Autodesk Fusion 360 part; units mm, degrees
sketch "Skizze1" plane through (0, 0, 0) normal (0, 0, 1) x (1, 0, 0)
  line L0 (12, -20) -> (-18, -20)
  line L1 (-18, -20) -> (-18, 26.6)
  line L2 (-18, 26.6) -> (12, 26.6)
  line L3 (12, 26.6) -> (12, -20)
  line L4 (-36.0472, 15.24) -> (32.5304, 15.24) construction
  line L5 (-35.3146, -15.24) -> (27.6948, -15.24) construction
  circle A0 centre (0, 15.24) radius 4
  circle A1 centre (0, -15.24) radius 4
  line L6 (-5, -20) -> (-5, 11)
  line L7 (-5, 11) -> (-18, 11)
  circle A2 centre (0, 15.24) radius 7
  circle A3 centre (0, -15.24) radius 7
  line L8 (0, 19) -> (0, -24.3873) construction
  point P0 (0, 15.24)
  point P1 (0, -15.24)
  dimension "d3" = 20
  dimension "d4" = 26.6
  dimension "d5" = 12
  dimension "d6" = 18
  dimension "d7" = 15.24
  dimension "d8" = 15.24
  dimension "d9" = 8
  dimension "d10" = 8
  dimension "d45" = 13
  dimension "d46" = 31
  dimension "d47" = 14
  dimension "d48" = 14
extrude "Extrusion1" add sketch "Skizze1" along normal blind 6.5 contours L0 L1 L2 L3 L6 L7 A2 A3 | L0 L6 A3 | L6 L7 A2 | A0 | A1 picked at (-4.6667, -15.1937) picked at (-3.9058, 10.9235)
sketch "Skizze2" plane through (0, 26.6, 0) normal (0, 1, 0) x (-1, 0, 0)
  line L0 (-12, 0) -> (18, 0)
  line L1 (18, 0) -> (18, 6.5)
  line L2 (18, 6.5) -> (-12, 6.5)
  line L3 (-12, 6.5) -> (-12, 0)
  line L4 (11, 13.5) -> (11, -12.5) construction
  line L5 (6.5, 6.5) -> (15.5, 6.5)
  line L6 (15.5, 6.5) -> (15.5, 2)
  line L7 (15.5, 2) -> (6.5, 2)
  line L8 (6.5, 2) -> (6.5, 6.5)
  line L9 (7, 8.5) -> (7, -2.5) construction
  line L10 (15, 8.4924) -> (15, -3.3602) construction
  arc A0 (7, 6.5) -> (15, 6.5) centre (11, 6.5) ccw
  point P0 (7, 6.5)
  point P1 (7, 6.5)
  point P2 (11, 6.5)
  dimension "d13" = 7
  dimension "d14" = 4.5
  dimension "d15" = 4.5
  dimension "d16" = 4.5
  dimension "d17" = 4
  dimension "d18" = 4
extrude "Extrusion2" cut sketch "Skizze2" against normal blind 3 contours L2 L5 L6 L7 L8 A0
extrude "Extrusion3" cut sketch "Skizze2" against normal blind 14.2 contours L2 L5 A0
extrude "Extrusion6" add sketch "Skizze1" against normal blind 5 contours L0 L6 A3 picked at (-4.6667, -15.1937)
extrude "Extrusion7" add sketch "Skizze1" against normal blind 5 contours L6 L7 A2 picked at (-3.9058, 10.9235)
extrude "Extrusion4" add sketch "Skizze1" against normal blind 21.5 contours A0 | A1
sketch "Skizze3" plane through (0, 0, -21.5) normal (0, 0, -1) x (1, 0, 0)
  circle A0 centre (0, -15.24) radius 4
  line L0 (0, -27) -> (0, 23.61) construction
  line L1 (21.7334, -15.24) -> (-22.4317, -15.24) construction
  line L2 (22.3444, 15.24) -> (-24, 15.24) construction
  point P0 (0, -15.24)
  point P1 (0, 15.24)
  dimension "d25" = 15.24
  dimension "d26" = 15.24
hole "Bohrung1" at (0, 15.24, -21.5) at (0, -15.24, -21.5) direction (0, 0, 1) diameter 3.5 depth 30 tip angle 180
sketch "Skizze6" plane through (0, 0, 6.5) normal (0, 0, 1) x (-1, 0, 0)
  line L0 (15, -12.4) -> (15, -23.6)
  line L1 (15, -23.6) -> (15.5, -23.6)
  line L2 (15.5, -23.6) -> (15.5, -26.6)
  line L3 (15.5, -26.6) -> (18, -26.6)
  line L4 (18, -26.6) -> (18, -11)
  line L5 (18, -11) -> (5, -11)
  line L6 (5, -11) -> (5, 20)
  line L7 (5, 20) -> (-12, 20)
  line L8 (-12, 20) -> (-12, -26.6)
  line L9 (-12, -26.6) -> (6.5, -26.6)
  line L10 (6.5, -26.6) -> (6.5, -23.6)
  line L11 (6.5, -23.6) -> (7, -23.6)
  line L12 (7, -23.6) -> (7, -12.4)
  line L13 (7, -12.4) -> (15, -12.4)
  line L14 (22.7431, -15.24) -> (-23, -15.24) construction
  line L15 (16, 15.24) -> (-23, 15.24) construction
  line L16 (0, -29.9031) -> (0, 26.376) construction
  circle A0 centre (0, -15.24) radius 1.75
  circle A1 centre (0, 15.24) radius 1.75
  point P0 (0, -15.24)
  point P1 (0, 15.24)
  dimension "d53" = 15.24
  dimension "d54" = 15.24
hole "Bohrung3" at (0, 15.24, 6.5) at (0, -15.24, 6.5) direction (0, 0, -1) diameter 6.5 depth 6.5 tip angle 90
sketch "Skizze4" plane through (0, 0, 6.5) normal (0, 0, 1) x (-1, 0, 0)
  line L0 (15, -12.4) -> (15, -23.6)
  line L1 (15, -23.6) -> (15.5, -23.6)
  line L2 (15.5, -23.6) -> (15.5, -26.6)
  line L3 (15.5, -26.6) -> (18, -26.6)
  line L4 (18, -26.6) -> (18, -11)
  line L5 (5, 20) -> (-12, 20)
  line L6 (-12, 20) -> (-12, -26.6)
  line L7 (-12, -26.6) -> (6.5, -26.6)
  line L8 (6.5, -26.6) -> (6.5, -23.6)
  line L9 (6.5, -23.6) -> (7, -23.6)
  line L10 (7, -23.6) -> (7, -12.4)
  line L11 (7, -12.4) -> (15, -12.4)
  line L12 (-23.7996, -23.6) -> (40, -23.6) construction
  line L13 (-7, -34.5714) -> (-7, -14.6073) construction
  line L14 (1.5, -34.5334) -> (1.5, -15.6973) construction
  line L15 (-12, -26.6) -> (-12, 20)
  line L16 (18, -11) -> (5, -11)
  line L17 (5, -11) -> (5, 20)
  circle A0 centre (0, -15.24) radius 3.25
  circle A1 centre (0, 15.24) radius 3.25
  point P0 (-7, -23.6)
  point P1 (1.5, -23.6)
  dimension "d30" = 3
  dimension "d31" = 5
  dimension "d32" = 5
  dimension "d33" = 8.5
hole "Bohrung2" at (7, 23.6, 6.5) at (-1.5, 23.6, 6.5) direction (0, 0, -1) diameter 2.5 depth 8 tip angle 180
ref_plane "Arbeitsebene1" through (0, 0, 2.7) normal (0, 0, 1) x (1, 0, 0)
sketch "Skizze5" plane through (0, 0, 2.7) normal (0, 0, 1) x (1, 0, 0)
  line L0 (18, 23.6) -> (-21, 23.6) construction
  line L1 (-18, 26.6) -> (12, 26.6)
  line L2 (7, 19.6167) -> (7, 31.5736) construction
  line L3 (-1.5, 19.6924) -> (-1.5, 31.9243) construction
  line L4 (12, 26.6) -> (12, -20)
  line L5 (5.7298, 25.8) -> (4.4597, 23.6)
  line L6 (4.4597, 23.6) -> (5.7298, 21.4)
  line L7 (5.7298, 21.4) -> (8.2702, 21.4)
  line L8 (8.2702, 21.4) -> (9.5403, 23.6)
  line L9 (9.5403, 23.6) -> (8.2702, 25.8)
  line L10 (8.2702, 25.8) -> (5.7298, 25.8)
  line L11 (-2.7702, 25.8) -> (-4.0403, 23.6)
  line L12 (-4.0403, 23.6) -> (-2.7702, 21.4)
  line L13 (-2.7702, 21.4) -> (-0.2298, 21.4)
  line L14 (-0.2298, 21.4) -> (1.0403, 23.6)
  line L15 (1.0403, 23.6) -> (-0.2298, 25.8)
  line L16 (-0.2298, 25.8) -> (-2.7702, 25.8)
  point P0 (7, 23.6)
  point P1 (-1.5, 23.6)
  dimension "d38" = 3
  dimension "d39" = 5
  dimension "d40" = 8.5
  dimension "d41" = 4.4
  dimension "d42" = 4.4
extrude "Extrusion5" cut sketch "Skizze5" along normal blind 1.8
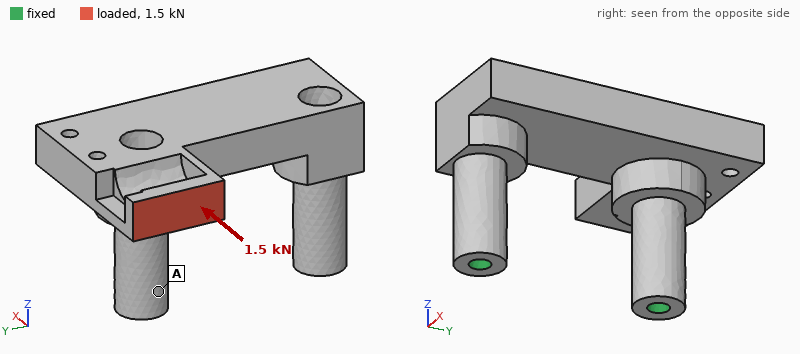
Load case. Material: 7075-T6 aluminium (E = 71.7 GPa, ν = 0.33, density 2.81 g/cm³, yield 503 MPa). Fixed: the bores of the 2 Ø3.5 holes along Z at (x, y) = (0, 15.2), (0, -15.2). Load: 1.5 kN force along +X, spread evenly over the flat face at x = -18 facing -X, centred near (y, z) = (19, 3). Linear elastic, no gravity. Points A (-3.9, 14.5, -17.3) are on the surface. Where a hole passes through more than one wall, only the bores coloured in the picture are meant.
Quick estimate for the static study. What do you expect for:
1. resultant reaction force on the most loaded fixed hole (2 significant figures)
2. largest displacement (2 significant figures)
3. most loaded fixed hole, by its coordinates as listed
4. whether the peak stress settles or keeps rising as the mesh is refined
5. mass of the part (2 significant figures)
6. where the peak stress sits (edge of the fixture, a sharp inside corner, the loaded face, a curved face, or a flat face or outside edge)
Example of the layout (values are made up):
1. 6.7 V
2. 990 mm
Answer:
1. 1.5 kN
2. 0.11 mm
3. (0, 15.2)
4. keeps rising
5. 23 g
6. edge of the fixture
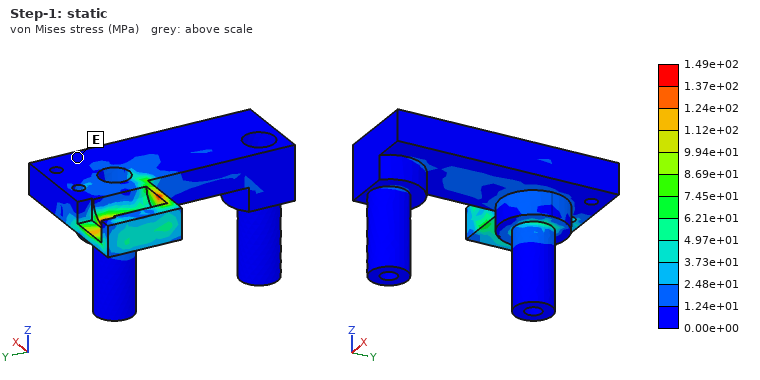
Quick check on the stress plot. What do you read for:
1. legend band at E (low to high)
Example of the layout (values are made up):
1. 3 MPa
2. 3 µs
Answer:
1. 0.00e+00 to 1.24e+01 MPa
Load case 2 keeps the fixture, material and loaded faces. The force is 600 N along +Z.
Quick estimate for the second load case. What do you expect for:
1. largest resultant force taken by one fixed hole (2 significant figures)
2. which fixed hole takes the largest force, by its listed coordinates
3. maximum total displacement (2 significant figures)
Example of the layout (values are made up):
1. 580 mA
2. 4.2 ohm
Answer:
1. 660 N
2. (0, 15.2)
3. 0.17 mm
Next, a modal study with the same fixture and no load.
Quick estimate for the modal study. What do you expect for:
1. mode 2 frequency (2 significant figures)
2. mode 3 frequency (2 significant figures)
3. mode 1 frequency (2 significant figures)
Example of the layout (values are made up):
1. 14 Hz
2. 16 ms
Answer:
1. 15 kHz
2. 17 kHz
3. 10 kHz
